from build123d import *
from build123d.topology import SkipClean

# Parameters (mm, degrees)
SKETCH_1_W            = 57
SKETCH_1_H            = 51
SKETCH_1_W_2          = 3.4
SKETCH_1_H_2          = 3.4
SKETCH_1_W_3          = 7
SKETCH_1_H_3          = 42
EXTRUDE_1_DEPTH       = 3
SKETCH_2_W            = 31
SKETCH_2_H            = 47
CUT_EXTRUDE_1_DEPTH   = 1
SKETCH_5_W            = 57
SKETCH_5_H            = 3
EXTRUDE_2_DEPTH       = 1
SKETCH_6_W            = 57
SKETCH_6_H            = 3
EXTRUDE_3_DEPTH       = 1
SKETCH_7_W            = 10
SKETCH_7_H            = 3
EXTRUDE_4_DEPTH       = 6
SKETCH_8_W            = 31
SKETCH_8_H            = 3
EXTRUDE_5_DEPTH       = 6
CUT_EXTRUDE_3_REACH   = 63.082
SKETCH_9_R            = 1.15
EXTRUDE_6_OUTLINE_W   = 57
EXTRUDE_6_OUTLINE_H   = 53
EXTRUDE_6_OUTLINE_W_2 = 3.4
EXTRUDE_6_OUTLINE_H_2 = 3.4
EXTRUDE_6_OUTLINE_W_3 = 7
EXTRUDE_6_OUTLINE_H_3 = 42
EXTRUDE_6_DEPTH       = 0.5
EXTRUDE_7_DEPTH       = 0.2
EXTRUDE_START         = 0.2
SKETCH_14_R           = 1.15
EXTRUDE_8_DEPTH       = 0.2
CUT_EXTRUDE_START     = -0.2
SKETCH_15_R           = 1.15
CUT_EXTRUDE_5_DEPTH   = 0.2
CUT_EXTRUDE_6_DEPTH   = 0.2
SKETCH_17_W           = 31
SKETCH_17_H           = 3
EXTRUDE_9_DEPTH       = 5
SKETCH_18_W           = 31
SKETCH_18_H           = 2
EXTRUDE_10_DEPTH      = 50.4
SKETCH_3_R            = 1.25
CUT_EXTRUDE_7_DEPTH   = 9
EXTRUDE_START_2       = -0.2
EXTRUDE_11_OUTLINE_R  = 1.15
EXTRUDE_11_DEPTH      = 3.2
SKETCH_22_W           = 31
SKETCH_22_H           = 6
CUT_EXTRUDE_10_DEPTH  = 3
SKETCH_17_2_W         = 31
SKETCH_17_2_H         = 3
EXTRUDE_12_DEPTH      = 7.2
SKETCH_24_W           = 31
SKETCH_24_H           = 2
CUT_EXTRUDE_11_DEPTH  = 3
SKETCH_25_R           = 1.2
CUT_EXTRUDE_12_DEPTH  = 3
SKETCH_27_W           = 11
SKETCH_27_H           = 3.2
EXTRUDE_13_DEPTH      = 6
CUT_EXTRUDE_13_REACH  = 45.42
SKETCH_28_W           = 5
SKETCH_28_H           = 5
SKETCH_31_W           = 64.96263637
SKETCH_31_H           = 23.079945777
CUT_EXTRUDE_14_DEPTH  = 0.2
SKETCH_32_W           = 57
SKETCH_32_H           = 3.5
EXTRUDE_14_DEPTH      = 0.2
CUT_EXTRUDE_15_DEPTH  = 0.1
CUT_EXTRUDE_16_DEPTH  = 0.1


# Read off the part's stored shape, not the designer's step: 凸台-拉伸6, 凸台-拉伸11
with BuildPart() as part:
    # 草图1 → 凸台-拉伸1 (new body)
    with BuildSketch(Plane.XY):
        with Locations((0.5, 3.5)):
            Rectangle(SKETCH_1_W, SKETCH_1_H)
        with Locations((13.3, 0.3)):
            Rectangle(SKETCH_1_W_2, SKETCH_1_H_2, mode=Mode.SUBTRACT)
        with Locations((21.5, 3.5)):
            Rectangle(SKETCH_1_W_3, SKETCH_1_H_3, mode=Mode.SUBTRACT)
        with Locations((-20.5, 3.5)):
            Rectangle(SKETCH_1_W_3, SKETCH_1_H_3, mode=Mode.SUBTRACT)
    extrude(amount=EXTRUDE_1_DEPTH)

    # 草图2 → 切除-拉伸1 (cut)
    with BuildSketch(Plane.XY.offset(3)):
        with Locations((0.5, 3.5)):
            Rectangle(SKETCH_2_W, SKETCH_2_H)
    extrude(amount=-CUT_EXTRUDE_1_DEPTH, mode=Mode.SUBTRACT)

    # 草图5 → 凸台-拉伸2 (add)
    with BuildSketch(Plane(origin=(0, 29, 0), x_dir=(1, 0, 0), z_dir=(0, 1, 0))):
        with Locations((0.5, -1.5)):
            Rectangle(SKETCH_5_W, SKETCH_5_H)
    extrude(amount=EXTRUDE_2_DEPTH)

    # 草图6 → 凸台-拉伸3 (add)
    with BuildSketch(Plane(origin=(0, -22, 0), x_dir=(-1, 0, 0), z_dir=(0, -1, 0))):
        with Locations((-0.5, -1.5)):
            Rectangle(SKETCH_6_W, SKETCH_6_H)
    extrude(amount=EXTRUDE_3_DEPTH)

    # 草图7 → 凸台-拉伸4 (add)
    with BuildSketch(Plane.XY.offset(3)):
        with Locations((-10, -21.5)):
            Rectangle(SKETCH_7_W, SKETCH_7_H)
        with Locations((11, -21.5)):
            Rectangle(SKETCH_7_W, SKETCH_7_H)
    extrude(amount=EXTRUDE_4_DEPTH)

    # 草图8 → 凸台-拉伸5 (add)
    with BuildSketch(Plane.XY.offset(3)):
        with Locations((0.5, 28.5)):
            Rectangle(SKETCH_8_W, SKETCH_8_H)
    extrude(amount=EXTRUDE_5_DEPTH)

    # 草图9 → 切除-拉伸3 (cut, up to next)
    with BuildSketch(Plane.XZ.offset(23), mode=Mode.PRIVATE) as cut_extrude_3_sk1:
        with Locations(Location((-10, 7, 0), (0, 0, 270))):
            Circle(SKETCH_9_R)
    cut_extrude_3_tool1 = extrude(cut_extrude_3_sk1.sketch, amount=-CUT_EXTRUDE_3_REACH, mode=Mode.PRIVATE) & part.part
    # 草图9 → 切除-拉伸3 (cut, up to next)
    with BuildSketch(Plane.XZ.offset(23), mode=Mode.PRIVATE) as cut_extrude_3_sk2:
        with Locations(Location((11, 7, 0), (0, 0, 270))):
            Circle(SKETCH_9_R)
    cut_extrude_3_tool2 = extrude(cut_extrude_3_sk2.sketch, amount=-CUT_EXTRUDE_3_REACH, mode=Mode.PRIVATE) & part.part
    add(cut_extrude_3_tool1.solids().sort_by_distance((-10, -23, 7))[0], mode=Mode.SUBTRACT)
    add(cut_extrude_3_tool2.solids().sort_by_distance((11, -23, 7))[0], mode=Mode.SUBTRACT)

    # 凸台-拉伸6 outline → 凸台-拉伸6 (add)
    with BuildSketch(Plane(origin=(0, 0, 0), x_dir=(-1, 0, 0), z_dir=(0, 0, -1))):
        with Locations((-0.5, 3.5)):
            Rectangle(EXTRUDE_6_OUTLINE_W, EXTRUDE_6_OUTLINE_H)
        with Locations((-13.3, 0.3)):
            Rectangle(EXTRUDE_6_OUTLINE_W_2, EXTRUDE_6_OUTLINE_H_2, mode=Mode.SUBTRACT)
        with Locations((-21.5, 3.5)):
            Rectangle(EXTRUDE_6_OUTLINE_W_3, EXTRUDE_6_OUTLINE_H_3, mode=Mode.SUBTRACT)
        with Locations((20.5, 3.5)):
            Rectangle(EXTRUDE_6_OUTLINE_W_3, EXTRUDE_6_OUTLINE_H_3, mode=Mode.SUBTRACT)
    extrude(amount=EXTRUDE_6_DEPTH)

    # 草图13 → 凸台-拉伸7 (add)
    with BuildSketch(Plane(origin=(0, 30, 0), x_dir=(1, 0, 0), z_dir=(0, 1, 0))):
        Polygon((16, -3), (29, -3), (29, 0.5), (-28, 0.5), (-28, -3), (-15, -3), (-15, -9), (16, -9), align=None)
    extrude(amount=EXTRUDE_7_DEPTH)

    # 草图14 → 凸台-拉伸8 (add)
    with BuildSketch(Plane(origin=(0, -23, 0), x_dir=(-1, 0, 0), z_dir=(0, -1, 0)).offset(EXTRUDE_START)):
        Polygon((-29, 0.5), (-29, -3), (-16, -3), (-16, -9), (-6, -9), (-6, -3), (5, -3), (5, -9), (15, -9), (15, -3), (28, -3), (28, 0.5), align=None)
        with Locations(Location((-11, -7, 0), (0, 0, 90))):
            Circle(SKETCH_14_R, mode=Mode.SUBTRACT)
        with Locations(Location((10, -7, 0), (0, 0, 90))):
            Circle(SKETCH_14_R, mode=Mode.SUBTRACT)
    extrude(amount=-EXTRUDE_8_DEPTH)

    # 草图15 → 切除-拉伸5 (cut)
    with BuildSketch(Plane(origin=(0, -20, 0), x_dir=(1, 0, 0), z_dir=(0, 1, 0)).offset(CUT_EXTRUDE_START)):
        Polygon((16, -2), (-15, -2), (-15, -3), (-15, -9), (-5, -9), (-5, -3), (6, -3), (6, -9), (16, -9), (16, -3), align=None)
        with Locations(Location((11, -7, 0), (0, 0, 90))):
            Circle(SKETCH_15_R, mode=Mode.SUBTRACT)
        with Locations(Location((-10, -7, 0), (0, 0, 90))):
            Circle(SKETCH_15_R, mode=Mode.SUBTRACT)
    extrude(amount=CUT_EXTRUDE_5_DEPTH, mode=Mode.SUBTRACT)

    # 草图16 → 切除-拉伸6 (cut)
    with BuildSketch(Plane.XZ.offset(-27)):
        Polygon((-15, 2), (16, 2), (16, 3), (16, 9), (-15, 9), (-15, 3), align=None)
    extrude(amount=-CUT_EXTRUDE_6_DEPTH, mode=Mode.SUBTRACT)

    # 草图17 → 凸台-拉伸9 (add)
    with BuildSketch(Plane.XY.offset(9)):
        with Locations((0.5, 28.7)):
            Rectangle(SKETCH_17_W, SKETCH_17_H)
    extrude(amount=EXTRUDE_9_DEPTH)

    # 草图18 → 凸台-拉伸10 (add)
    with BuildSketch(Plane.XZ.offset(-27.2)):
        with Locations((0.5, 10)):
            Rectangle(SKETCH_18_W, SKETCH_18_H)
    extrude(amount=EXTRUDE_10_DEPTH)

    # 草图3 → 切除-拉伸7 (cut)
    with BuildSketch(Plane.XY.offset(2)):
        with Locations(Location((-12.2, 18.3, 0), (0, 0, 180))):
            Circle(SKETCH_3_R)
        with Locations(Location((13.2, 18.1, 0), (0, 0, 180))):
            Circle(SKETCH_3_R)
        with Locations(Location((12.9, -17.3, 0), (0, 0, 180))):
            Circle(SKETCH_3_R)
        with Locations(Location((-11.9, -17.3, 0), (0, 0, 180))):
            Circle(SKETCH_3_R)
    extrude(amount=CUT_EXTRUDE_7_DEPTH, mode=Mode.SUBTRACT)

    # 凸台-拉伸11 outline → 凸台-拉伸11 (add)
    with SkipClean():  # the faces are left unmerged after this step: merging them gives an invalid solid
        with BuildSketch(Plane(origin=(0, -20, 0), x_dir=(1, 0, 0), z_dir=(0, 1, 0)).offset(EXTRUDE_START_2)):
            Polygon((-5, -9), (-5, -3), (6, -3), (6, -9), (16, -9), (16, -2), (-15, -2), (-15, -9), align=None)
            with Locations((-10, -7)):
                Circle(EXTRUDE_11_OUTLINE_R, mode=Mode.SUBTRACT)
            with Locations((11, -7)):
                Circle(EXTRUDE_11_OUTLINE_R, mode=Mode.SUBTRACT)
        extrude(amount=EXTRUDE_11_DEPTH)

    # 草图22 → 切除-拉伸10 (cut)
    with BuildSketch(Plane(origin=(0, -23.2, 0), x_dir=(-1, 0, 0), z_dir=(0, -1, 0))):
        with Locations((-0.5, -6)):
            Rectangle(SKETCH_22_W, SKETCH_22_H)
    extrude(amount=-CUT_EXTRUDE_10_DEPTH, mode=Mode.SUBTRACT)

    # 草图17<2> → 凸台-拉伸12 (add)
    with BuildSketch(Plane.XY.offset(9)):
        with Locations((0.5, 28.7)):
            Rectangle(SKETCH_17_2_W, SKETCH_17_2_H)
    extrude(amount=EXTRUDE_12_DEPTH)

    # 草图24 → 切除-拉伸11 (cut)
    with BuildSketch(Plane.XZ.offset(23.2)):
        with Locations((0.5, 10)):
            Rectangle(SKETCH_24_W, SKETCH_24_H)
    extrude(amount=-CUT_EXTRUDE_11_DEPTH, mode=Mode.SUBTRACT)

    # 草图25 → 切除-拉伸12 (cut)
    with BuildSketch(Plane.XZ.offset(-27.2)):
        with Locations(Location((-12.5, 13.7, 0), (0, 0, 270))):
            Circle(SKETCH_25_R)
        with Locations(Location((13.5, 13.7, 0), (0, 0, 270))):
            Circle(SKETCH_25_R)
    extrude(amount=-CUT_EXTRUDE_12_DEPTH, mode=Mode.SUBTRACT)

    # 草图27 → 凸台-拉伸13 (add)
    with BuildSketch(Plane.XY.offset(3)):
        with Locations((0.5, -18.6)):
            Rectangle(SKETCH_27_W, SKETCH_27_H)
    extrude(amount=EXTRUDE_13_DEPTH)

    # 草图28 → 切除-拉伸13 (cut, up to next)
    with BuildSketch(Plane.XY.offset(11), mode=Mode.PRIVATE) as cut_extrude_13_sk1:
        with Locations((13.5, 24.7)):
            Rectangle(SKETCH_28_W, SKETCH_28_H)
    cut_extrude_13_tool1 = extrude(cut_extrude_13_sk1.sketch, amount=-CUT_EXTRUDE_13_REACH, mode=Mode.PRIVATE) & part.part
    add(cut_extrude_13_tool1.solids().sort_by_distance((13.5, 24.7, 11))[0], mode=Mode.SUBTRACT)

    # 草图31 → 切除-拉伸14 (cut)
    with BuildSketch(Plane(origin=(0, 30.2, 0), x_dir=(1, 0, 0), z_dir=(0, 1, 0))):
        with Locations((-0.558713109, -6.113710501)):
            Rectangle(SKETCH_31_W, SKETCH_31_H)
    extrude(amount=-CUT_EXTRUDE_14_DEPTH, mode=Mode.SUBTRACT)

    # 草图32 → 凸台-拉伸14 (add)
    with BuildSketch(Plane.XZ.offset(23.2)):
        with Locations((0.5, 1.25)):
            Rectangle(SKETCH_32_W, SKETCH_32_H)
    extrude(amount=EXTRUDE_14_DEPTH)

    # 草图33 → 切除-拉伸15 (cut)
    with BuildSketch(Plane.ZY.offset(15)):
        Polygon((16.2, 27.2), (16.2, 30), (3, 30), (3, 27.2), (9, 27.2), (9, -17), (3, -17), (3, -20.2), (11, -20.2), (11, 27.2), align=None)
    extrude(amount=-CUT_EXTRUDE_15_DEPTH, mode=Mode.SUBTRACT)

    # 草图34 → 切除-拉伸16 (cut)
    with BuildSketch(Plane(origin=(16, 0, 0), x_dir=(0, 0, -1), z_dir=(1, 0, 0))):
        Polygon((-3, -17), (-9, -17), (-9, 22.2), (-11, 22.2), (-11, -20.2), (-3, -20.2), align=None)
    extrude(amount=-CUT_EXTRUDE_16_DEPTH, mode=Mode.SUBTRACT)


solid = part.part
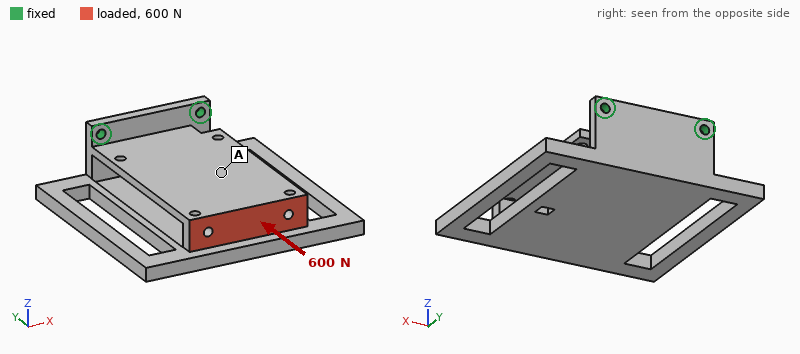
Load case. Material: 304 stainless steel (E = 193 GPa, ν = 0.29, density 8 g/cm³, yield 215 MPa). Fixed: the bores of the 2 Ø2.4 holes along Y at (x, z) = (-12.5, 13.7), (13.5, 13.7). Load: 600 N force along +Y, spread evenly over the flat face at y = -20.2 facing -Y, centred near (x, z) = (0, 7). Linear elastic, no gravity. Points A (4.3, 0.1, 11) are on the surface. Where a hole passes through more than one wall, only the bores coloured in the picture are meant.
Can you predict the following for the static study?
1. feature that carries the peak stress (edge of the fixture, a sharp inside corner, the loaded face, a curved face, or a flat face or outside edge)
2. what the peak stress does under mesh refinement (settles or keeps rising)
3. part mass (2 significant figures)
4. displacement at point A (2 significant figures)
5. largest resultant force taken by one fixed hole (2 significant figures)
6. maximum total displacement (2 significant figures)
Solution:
edge of the fixture
keeps rising
94 g
0.057 mm
320 N
0.11 mm
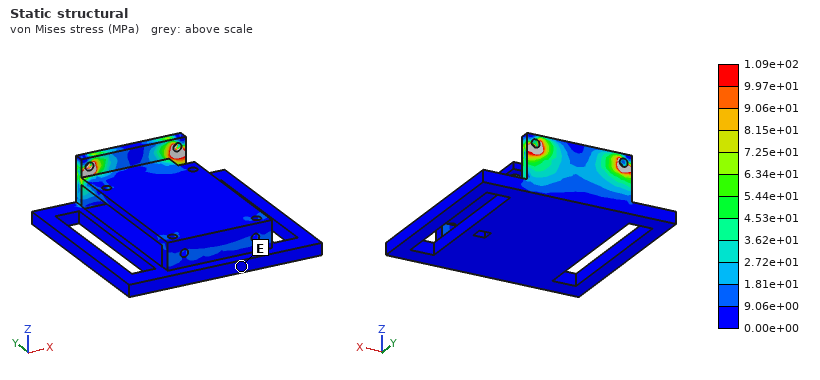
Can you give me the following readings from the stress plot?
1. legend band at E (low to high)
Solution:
0.00e+00 to 9.06e+00 MPa
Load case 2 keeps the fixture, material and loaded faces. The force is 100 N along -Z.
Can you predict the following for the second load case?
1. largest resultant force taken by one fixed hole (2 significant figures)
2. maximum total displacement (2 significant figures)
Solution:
56 N
0.28 mm
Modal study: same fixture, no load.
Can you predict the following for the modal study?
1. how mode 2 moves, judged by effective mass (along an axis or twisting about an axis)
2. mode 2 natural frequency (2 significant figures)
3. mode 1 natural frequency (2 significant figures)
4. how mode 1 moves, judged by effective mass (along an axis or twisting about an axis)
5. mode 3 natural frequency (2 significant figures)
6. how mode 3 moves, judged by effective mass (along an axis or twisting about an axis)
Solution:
along X
1800 Hz
510 Hz
along Z
2500 Hz
along X
